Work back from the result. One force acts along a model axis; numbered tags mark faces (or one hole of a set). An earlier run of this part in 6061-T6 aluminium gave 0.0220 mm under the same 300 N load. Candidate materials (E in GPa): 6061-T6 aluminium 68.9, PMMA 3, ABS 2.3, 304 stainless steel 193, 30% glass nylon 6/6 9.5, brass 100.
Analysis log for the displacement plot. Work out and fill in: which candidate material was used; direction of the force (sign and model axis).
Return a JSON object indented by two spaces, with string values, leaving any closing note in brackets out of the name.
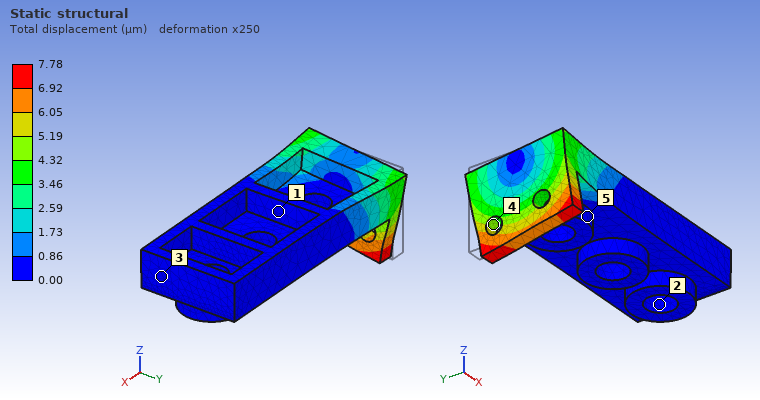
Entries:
{
  "which candidate material was used": "304 stainless steel",
  "direction of the force": "-Y"
}
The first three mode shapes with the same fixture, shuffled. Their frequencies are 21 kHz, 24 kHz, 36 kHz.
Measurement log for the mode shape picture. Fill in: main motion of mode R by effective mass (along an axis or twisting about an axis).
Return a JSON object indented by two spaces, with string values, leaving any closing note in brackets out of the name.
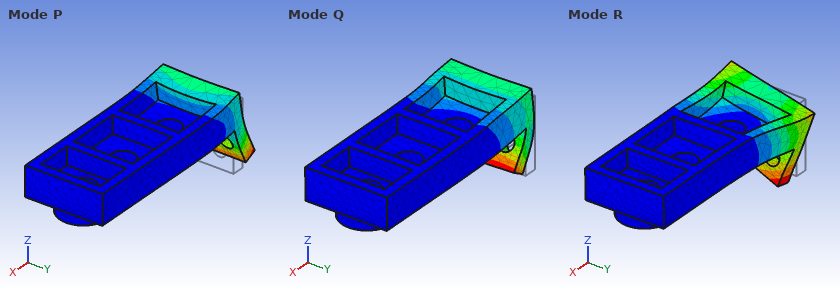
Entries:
{
  "main motion of mode R by effective mass": "twisting about X"
}
